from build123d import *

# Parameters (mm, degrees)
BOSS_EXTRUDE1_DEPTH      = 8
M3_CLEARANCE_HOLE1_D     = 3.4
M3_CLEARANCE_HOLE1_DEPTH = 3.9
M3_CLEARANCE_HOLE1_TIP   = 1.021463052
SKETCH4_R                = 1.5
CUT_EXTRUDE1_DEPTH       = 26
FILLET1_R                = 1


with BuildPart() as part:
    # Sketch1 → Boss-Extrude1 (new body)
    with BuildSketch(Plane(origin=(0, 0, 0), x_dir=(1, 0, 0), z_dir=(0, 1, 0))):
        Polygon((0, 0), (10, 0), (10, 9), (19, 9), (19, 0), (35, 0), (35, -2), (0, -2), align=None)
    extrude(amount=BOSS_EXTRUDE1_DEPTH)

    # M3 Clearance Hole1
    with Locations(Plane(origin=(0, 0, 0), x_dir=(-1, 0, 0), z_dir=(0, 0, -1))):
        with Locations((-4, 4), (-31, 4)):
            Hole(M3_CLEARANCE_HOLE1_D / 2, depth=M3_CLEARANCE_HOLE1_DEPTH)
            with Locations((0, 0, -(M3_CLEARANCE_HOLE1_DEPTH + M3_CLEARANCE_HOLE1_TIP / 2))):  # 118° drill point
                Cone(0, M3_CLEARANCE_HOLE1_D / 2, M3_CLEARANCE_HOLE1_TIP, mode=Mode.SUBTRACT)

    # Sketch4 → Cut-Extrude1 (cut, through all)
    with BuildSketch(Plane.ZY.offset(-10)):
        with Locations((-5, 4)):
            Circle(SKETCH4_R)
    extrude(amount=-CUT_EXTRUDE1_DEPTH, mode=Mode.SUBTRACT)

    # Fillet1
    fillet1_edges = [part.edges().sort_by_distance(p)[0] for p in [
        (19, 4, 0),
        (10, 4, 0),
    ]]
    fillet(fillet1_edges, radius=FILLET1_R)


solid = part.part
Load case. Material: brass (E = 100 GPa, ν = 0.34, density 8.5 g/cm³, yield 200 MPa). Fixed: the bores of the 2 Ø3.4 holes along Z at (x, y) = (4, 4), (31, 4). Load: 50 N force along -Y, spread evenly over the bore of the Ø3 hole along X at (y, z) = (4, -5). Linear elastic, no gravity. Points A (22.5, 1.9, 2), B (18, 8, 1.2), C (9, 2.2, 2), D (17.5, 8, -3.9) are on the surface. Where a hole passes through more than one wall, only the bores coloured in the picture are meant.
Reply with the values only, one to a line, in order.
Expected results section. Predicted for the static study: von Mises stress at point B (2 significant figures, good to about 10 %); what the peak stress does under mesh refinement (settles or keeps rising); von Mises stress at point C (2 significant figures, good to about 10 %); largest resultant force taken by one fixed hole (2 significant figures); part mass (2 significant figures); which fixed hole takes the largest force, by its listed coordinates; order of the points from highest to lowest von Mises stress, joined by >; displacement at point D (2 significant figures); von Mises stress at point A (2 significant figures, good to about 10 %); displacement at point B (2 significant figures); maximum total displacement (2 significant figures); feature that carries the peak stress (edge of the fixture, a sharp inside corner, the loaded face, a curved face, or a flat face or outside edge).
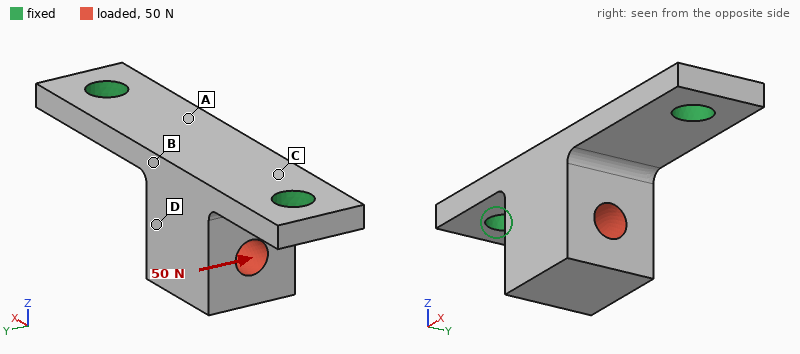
6.8 MPa
keeps rising
18 MPa
34 N
9.4 g
(4, 4)
C > A > B > D
8.2 µm
11 MPa
4.6 µm
13 µm
edge of the fixture
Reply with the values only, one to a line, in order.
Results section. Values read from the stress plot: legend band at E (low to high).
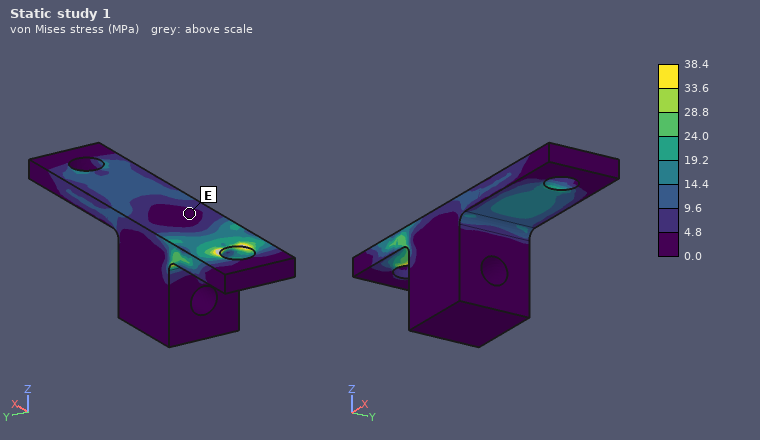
0.0 to 4.8 MPa
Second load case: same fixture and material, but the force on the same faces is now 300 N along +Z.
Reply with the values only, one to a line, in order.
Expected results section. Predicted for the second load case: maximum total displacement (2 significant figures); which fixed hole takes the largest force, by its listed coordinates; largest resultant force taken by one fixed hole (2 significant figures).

26 µm
(4, 4)
200 N
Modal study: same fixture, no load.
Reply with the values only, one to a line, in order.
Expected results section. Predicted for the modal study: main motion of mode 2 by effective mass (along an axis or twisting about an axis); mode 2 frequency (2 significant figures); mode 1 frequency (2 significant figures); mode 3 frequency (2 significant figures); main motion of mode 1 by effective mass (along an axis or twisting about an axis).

along Z
7000 Hz
5200 Hz
15 kHz
along Y
